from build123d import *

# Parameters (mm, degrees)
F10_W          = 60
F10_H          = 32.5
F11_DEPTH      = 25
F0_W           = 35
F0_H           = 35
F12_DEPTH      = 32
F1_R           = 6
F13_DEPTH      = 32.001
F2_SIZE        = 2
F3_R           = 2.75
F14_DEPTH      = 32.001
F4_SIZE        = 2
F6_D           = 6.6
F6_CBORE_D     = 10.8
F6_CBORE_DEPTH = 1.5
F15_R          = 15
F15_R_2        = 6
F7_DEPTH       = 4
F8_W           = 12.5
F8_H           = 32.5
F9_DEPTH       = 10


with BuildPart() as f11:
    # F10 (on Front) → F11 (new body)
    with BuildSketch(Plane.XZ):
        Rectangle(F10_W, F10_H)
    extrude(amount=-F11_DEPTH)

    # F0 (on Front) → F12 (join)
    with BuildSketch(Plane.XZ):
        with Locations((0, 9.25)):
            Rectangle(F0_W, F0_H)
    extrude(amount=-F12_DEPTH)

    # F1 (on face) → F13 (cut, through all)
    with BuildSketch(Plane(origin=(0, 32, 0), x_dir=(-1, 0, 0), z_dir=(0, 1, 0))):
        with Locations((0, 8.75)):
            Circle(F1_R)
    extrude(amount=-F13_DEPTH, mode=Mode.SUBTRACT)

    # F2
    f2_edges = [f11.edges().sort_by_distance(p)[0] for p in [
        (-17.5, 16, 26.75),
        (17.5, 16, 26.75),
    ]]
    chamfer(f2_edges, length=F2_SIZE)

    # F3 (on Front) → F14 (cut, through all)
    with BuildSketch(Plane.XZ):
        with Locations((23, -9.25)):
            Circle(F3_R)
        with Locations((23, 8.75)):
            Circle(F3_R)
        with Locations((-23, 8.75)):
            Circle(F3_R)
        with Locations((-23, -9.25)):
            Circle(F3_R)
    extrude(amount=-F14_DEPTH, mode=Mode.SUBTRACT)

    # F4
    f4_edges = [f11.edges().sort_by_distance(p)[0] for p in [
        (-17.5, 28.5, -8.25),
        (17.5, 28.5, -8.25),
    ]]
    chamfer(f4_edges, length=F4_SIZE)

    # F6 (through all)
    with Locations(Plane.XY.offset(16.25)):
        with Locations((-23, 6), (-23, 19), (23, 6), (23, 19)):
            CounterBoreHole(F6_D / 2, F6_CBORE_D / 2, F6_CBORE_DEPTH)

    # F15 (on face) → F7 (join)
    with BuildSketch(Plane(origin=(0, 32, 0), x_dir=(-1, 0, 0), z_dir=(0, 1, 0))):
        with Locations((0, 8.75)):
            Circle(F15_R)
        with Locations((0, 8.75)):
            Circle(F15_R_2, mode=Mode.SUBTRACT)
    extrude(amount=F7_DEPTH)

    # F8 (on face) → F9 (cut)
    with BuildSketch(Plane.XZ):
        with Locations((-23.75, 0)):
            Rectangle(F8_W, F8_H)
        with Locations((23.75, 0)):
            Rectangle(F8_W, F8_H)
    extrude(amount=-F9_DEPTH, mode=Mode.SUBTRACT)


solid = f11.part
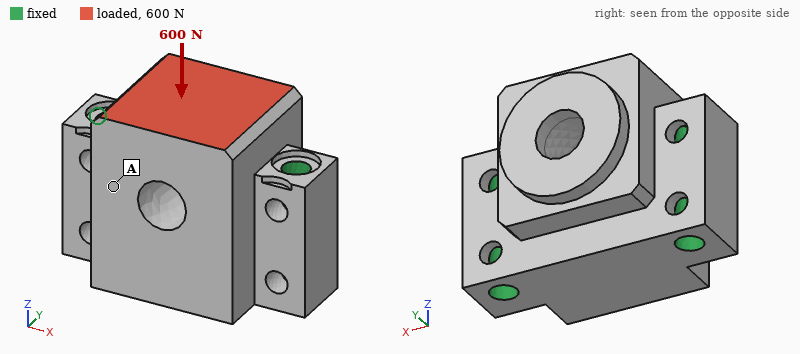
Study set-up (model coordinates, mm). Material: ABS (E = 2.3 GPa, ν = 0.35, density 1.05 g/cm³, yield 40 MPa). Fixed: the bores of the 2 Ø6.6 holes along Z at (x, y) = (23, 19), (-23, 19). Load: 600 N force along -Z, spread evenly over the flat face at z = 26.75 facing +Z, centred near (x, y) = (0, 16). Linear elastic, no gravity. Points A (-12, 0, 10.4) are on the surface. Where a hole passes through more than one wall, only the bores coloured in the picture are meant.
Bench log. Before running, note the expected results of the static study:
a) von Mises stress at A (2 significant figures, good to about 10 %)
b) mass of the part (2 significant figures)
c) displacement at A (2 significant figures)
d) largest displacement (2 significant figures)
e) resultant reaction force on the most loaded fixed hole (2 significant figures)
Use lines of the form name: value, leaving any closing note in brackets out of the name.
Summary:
von Mises stress at A: 0.48 MPa
mass of the part: 56 g
displacement at A: 14 µm
largest displacement: 22 µm
resultant reaction force on the most loaded fixed hole: 310 N
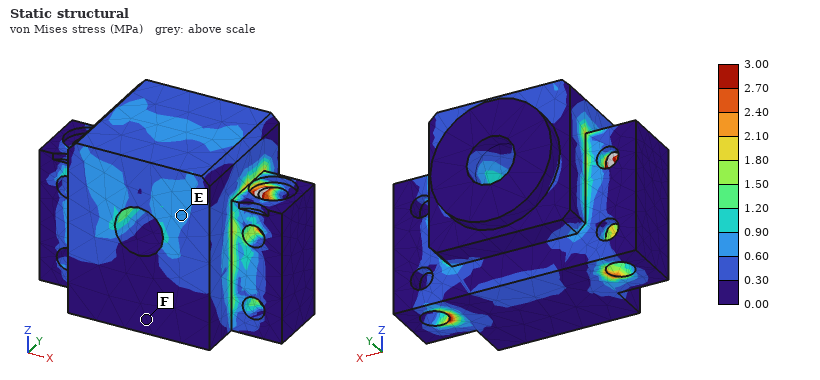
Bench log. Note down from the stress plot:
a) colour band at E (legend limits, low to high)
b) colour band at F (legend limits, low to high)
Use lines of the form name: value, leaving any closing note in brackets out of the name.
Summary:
colour band at E: 0.60 to 0.90 MPa
colour band at F: 0.00 to 0.30 MPa
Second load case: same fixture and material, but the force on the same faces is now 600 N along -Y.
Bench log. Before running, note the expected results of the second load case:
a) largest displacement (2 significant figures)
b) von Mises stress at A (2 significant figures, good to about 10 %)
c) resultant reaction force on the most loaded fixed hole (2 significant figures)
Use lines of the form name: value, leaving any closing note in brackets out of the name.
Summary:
largest displacement: 0.10 mm
von Mises stress at A: 1.9 MPa
resultant reaction force on the most loaded fixed hole: 300 N
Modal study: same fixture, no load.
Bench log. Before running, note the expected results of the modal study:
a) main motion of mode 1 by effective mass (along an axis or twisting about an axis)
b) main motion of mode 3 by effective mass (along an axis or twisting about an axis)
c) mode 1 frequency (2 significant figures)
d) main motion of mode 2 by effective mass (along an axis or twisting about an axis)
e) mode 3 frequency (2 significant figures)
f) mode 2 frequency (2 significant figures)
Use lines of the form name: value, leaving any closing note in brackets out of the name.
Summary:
main motion of mode 1 by effective mass: along Y
main motion of mode 3 by effective mass: along Y
mode 1 frequency: 3700 Hz
main motion of mode 2 by effective mass: along Z
mode 3 frequency: 6800 Hz
mode 2 frequency: 6100 Hz
